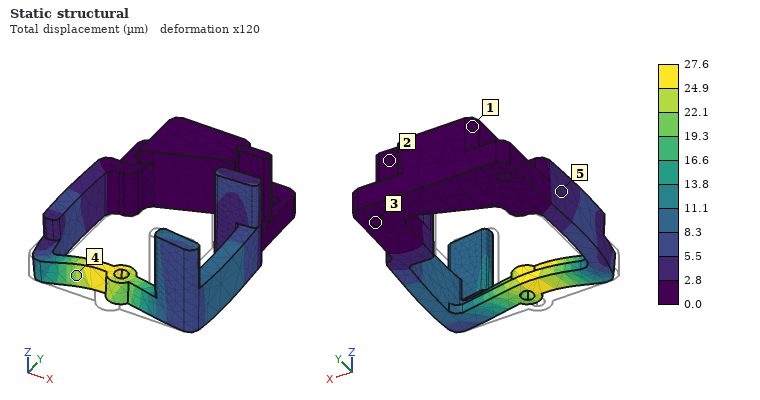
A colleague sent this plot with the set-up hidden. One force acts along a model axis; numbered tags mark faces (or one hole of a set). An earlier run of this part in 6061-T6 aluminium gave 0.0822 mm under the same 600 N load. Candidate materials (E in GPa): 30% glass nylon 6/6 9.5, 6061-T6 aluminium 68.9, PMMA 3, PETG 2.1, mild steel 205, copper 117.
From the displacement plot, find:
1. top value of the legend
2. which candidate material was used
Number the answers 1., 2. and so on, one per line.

1. 27.6 µm
2. mild steel
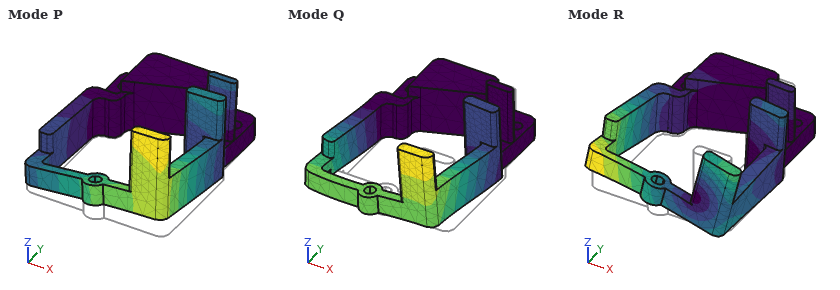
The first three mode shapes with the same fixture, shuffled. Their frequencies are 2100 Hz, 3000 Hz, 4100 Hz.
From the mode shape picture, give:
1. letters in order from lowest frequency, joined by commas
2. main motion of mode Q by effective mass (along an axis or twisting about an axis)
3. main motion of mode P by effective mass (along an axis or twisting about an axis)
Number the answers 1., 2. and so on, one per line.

1. P, Q, R
2. along X
3. along Z
